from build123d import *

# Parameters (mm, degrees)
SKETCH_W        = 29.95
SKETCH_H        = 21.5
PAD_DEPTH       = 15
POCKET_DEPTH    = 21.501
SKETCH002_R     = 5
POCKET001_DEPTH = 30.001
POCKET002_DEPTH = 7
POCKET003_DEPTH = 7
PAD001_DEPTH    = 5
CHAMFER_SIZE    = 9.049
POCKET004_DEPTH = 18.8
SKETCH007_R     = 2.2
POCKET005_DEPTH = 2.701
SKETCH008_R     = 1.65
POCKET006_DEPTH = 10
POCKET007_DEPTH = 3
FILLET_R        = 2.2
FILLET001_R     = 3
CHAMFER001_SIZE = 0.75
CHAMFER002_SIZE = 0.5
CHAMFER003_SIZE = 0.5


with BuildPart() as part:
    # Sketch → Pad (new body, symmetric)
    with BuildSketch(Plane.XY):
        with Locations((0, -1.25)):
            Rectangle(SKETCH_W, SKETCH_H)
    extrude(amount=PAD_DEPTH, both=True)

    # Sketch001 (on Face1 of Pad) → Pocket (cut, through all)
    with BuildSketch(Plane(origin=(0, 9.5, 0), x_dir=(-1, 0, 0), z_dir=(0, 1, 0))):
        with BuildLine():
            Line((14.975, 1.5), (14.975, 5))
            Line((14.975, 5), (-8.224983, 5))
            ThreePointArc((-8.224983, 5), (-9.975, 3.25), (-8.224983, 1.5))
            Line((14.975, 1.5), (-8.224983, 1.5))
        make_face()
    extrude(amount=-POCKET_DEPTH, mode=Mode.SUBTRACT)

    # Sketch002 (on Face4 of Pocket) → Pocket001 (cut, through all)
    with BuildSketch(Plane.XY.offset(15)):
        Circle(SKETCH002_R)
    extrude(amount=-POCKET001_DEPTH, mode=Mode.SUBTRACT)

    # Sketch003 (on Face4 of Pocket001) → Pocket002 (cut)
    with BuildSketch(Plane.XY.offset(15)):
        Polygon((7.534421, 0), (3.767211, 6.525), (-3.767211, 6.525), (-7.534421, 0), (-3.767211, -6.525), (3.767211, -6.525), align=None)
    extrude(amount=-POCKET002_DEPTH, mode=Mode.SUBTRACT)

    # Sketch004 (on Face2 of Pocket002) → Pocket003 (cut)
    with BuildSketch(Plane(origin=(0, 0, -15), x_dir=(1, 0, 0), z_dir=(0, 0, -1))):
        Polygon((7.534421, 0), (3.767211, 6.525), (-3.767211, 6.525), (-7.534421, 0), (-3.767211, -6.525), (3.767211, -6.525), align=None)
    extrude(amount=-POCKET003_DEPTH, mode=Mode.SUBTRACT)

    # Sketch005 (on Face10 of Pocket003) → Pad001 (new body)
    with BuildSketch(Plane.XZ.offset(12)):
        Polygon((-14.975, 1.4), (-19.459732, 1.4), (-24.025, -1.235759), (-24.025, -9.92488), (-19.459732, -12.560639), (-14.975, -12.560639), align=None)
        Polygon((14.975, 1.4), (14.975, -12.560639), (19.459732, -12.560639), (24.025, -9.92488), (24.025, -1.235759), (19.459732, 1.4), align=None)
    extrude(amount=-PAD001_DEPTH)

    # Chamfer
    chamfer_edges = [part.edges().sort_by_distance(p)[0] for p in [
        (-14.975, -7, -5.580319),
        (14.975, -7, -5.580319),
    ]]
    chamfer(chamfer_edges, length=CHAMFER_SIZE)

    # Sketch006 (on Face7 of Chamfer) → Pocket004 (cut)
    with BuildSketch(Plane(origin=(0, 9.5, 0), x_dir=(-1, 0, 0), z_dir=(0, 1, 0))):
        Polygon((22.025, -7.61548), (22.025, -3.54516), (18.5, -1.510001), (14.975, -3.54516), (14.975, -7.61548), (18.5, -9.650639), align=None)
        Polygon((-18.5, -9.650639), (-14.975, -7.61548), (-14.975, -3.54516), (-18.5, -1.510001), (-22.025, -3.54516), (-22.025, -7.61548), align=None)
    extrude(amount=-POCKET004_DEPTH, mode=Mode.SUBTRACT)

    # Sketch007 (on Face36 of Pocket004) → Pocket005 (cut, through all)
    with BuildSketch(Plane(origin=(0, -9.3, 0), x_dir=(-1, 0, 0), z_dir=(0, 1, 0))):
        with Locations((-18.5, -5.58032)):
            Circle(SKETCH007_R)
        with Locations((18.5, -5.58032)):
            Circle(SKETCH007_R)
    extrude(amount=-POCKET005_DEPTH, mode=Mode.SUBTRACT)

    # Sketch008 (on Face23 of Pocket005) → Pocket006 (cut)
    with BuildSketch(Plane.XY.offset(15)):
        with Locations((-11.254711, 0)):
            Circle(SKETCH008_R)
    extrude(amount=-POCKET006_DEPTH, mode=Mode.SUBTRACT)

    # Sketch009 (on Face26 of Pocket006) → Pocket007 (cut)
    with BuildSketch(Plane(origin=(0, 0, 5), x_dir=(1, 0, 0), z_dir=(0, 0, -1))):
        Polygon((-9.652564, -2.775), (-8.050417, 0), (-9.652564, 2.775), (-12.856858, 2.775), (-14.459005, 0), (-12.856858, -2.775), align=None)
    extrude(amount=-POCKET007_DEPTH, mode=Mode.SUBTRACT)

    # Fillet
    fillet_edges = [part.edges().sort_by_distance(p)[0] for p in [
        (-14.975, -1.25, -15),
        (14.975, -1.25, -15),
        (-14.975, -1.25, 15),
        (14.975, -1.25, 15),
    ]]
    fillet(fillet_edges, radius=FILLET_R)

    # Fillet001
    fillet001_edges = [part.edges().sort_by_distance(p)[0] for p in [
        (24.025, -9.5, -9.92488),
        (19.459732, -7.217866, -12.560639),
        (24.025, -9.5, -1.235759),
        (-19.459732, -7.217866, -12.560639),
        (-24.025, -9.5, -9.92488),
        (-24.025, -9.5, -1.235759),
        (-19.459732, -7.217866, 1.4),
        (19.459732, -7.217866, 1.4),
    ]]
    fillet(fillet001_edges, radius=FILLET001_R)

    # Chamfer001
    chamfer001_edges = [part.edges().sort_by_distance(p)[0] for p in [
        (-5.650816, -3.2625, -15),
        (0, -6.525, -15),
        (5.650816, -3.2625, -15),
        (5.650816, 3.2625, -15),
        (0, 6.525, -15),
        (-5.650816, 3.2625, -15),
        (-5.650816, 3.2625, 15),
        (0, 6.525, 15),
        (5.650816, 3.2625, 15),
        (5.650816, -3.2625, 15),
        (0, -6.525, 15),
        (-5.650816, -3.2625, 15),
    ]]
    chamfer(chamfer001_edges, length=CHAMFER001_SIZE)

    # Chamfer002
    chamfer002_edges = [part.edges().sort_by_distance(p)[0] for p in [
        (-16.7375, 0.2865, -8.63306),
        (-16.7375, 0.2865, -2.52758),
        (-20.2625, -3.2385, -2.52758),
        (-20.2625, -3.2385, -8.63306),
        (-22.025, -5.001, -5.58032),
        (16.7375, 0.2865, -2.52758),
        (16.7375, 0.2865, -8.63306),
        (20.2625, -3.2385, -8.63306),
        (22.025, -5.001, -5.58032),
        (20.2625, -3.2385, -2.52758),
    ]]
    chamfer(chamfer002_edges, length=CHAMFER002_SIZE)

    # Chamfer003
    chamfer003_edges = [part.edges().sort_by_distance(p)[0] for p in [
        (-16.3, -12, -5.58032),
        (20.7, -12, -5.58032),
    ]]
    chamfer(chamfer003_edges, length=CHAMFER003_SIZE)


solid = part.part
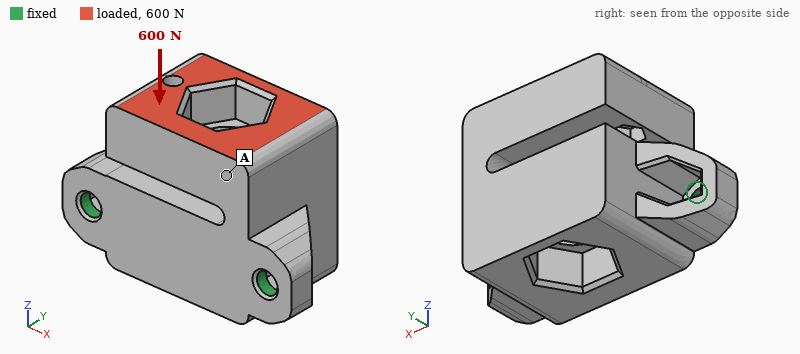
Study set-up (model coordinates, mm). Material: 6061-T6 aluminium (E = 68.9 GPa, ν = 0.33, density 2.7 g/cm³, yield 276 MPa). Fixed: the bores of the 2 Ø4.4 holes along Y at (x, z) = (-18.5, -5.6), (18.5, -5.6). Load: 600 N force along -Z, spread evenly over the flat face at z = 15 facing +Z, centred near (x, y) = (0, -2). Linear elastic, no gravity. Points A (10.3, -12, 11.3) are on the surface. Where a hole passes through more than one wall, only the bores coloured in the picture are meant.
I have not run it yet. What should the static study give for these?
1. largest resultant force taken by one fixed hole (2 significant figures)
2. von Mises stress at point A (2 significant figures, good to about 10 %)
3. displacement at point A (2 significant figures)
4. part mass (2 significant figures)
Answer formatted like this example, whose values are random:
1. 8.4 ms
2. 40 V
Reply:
1. 310 N
2. 17 MPa
3. 0.038 mm
4. 42 g
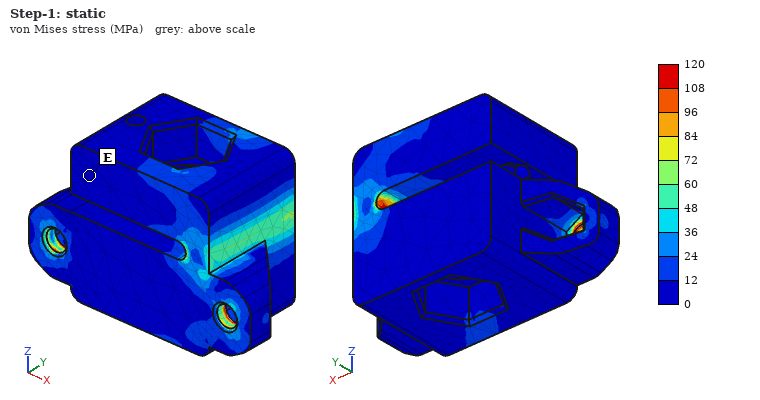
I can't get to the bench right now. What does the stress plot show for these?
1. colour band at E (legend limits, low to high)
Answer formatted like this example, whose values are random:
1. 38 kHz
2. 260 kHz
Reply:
1. 0 to 12 MPa
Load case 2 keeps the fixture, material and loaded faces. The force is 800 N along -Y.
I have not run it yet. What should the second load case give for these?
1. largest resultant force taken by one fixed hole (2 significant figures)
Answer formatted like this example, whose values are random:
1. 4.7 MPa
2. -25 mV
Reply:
1. 540 N
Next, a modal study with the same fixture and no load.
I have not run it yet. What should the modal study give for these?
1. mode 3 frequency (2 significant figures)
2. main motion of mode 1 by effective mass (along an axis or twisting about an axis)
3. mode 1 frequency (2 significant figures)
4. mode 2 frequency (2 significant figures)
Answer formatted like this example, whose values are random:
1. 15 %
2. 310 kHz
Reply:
1. 6900 Hz
2. along Z
3. 2900 Hz
4. 3700 Hz
